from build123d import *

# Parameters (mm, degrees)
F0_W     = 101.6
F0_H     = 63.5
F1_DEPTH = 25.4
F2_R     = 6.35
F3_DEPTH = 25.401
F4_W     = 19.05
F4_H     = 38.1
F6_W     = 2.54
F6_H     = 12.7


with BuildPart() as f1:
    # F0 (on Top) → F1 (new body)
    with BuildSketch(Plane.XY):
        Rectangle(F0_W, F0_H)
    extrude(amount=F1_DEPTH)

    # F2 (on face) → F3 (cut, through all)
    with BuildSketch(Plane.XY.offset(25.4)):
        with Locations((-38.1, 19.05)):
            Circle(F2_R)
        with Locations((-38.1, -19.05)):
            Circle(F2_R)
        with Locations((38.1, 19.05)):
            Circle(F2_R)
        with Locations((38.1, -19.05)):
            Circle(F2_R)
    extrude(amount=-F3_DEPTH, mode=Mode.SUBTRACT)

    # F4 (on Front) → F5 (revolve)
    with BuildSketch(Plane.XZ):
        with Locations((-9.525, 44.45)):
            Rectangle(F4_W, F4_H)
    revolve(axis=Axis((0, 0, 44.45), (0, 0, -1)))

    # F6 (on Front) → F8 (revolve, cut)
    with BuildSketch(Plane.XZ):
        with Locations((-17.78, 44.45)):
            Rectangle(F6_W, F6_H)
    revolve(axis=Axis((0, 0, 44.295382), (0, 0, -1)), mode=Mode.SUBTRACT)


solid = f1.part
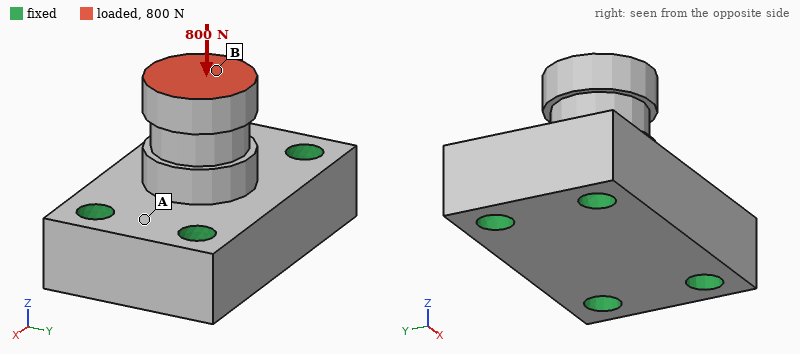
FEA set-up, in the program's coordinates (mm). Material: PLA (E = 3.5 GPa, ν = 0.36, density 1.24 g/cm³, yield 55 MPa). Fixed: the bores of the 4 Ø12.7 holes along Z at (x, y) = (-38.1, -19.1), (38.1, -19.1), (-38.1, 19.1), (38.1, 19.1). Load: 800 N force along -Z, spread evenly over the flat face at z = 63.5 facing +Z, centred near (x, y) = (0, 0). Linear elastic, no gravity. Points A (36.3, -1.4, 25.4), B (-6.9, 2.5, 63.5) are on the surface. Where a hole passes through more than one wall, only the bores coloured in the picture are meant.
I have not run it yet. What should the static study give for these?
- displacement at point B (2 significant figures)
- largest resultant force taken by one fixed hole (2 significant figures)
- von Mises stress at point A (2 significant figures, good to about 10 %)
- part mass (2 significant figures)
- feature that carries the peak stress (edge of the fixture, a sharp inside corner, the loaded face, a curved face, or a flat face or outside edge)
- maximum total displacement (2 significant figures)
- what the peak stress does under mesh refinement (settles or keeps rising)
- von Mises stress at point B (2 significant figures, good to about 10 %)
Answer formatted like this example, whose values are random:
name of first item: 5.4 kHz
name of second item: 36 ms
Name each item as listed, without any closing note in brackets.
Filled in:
displacement at point B: 17 µm
largest resultant force taken by one fixed hole: 210 N
von Mises stress at point A: 0.21 MPa
part mass: 240 g
feature that carries the peak stress: edge of the fixture
maximum total displacement: 18 µm
what the peak stress does under mesh refinement: keeps rising
von Mises stress at point B: 0.87 MPa
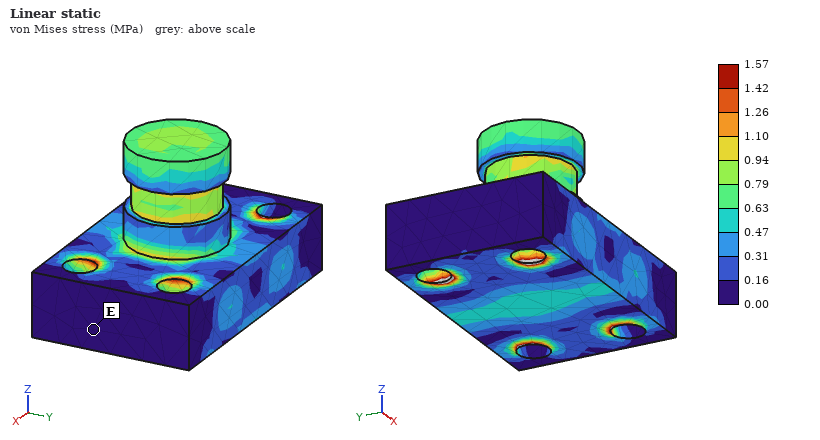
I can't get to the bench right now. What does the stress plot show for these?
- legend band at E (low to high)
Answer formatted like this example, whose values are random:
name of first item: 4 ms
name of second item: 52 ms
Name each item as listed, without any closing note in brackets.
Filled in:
legend band at E: 0.00 to 0.16 MPa
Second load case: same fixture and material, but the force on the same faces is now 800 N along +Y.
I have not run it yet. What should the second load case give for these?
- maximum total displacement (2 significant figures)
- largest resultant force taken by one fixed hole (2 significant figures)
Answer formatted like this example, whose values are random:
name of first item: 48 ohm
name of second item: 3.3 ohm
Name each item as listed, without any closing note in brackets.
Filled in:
maximum total displacement: 0.16 mm
largest resultant force taken by one fixed hole: 500 N
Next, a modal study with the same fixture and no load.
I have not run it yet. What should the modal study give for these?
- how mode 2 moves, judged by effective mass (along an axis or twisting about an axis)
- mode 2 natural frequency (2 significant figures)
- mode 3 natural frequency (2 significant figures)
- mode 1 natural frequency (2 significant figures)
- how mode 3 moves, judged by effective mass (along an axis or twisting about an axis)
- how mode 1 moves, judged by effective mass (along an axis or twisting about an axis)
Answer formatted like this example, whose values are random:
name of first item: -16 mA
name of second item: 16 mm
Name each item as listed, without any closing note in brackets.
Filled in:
how mode 2 moves, judged by effective mass: along X
mode 2 natural frequency: 3100 Hz
mode 3 natural frequency: 4300 Hz
mode 1 natural frequency: 2600 Hz
how mode 3 moves, judged by effective mass: along Z
how mode 1 moves, judged by effective mass: along Y
